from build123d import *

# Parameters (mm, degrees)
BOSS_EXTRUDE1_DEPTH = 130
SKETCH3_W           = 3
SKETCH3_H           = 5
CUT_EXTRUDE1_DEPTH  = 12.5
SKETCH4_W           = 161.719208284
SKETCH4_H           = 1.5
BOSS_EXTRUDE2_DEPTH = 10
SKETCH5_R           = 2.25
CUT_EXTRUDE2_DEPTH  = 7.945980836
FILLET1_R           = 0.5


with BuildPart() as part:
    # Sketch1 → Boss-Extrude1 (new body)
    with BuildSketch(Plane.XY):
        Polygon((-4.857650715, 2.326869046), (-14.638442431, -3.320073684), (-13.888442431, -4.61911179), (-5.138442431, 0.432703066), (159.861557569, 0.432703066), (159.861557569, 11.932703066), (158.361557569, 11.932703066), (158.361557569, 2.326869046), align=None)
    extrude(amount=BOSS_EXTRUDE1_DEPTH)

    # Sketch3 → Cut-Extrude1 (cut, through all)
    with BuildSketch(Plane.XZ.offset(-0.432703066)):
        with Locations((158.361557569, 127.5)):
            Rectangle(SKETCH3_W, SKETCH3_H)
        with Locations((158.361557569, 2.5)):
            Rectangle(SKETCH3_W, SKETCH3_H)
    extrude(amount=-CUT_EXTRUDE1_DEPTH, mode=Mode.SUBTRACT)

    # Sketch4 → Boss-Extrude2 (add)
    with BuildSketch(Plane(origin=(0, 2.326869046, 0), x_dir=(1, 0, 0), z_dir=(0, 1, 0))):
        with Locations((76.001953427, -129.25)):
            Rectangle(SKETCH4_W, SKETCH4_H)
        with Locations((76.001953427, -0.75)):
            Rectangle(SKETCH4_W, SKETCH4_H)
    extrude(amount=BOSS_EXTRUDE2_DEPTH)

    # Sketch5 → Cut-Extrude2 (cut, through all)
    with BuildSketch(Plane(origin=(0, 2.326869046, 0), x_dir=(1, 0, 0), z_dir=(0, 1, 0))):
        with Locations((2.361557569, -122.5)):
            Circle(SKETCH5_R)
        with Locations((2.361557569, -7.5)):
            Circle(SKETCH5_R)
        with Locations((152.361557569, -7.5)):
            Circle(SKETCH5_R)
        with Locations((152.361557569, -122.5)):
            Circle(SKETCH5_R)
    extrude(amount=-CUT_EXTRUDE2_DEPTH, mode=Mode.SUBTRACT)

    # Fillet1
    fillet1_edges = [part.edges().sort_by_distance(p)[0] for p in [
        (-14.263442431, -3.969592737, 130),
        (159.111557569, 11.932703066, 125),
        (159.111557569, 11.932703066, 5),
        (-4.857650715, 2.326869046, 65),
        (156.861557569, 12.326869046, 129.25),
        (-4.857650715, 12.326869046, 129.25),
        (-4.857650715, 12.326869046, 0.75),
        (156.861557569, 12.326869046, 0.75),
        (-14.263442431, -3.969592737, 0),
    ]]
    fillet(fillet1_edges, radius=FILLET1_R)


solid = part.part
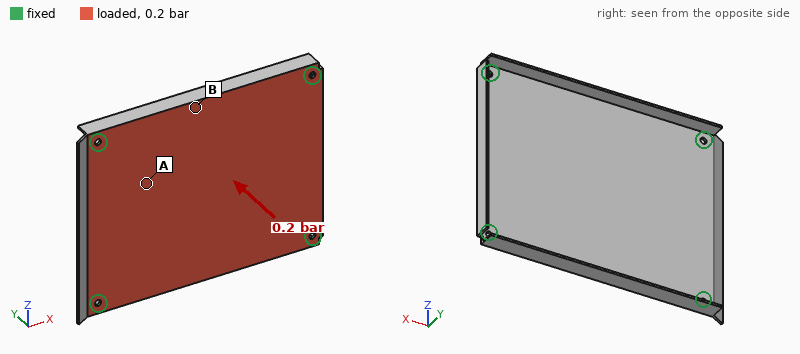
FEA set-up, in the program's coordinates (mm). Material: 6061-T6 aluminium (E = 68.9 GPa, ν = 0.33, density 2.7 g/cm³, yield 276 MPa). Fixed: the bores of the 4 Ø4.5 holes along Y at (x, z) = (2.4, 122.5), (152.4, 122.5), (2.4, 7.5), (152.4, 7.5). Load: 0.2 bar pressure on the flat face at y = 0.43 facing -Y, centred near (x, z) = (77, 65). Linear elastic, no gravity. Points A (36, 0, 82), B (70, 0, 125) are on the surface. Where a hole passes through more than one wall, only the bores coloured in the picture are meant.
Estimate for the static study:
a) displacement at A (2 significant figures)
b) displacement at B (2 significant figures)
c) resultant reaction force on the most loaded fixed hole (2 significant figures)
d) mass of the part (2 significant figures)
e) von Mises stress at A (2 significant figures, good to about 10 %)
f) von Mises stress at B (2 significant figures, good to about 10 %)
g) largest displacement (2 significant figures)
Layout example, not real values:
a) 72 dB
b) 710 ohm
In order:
a) 0.46 mm
b) 0.15 mm
c) 190 N
d) 130 g
e) 20 MPa
f) 7.9 MPa
g) 0.68 mm
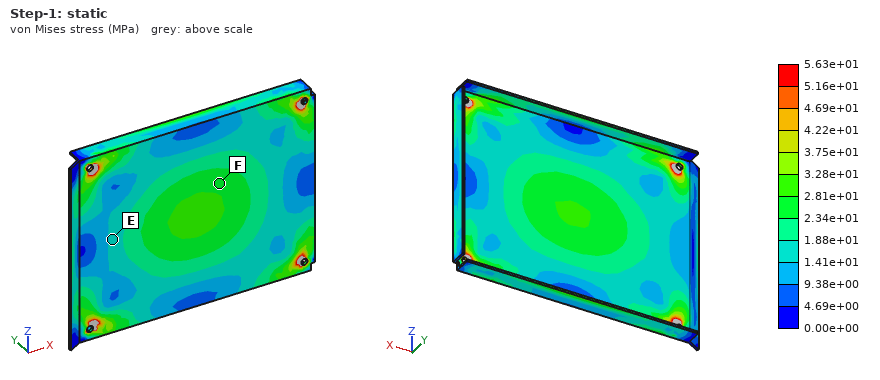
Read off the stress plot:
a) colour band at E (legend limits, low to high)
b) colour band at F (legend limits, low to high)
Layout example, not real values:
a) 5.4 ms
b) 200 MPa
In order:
a) 1.41e+01 to 1.88e+01 MPa
b) 2.34e+01 to 2.81e+01 MPa
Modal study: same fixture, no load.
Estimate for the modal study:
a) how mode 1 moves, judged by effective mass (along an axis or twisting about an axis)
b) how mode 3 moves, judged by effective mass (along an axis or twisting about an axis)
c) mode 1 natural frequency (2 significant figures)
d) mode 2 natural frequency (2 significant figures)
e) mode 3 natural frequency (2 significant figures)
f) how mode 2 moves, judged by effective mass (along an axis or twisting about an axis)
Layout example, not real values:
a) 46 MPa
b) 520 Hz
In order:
a) along Y
b) twisting about X
c) 480 Hz
d) 980 Hz
e) 1100 Hz
f) twisting about Z
